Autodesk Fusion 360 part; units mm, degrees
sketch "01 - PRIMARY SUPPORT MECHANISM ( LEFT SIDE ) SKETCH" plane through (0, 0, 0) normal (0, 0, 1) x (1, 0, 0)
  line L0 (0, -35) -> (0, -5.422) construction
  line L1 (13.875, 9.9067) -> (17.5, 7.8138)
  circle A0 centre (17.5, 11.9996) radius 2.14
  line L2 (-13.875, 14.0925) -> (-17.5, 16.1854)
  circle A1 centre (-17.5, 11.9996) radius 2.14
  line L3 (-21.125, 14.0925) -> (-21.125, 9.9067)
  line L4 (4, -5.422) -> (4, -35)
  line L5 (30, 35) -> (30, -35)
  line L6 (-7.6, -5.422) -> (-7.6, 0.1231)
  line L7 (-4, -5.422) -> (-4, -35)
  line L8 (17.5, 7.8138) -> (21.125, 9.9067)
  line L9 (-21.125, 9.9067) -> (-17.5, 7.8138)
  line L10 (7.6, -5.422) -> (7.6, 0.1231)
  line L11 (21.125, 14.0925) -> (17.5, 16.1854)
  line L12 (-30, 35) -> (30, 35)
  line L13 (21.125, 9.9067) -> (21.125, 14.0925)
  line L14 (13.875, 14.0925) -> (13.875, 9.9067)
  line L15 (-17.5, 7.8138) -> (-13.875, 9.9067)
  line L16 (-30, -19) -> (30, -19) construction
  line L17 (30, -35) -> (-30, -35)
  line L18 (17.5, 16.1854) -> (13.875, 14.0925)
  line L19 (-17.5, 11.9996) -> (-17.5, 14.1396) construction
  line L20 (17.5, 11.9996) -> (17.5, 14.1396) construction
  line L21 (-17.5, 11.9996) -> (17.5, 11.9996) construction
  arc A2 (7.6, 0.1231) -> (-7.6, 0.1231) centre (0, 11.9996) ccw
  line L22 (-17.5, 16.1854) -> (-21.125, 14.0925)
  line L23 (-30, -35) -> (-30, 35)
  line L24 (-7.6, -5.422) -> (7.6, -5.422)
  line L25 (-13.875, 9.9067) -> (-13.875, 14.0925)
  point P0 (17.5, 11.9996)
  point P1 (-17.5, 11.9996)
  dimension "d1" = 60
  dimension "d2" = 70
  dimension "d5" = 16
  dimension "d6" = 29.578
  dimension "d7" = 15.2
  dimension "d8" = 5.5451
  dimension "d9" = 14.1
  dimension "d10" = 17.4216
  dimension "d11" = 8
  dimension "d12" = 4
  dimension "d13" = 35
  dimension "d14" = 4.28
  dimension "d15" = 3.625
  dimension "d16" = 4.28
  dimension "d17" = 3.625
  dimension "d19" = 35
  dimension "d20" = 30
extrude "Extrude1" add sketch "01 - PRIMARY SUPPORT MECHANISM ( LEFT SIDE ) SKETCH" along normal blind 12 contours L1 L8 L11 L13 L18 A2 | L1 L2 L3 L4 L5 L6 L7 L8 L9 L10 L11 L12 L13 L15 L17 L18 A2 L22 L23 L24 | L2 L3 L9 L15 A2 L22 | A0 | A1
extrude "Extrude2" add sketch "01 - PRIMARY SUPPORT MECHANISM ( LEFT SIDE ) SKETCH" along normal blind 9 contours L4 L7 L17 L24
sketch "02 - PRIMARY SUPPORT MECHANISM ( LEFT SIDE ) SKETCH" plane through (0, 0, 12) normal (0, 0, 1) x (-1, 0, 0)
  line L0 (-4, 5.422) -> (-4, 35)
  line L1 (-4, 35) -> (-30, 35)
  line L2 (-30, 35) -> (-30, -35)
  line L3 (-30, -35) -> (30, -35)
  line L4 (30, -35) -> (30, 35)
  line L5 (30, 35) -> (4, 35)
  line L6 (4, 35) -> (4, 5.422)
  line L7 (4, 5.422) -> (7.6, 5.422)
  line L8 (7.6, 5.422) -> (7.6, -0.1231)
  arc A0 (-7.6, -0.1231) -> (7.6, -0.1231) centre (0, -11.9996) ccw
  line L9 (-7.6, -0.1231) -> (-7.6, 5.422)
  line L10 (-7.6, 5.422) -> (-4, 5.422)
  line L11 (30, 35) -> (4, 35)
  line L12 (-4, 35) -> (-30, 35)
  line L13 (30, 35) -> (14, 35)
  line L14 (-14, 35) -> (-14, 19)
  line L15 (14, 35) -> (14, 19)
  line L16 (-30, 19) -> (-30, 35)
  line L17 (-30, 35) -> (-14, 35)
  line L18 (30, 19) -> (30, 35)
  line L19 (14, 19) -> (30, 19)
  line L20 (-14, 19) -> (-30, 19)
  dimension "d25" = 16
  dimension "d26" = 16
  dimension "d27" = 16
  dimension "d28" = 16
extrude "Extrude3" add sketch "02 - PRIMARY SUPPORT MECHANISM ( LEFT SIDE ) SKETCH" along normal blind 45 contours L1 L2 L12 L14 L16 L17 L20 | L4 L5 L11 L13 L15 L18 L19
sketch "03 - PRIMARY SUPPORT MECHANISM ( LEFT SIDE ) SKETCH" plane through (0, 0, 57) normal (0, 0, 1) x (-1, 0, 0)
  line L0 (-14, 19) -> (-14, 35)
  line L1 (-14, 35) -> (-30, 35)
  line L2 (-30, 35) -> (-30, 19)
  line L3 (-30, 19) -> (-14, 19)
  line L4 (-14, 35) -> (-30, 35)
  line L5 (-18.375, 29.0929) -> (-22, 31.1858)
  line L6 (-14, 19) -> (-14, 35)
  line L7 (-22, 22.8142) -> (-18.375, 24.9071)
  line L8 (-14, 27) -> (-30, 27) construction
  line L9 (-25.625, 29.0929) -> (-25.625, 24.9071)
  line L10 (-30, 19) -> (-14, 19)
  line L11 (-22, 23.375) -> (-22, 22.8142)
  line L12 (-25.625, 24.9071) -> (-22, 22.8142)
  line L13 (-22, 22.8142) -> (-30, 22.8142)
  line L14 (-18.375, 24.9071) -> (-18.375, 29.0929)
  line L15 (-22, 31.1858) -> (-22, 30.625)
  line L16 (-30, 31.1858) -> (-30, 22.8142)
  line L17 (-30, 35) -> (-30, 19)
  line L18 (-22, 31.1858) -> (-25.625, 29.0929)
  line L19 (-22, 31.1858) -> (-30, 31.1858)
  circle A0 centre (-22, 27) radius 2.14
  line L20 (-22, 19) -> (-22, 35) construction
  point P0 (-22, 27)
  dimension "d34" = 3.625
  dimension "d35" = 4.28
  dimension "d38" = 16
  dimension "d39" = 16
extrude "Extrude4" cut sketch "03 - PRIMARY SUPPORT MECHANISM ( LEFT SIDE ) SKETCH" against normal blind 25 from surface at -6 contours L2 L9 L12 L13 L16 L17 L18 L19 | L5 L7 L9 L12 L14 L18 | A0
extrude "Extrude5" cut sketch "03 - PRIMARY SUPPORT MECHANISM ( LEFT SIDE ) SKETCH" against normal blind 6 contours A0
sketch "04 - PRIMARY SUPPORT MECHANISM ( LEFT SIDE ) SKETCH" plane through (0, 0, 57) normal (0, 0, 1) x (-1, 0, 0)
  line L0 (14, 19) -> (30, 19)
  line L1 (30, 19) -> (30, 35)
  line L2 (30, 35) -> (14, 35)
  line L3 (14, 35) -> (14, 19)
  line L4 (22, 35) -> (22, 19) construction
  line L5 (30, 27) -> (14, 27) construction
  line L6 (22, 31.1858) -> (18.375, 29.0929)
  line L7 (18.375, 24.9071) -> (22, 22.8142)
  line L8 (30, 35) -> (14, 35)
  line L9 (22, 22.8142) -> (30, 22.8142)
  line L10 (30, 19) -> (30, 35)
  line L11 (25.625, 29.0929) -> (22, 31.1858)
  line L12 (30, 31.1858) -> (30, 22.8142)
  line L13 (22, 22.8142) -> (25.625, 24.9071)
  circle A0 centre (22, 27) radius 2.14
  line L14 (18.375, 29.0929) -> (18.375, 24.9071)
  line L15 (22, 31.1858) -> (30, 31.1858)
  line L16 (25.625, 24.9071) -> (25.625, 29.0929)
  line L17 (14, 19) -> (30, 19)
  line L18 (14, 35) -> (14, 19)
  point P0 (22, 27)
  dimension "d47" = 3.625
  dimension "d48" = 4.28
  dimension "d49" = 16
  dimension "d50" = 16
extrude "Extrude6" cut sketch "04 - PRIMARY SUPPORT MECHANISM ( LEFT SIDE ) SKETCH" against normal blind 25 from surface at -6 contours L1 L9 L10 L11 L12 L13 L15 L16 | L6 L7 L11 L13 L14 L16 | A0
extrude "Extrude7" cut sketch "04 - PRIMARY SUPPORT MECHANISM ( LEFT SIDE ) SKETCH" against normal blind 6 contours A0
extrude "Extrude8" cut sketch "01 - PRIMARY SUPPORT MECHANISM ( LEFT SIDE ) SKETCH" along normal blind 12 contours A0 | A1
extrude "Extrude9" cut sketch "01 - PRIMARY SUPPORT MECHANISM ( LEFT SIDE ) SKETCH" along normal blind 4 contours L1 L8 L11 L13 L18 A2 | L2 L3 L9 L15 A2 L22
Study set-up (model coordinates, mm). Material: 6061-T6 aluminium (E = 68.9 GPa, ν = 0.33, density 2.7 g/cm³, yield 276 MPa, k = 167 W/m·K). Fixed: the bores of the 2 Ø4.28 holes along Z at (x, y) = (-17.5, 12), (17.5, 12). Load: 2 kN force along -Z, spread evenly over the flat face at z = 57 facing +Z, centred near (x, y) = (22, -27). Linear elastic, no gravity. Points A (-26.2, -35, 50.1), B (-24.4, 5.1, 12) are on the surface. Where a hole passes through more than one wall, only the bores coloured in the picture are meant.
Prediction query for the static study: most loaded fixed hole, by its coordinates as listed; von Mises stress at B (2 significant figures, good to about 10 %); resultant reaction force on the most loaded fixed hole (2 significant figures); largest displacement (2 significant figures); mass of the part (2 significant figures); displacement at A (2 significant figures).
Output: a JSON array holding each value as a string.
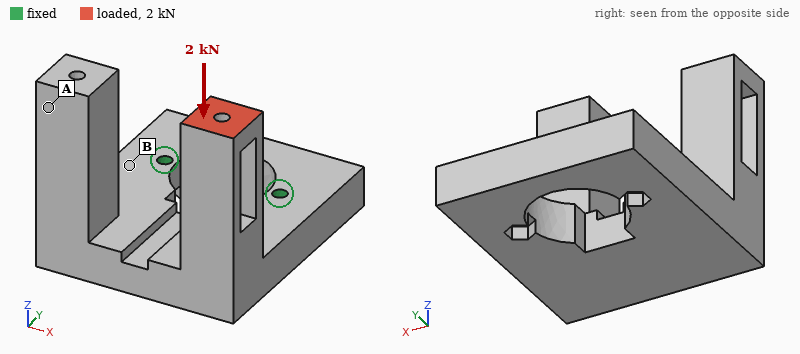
["(17.5, 12)", "57 MPa", "1.9 kN", "0.52 mm", "160 g", "0.31 mm"]
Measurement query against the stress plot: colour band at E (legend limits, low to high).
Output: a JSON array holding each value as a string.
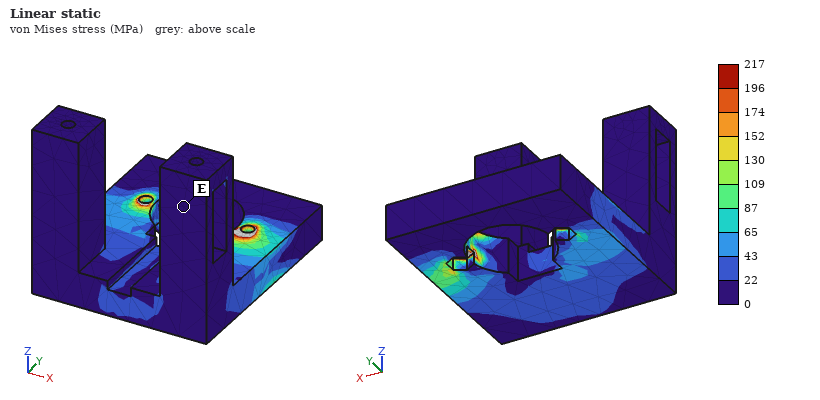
["0 to 22 MPa"]
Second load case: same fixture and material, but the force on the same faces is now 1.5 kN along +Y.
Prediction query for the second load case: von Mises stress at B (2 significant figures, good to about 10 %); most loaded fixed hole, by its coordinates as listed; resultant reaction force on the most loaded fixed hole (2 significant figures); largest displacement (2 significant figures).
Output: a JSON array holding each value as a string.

["72 MPa", "(17.5, 12)", "1.7 kN", "0.92 mm"]
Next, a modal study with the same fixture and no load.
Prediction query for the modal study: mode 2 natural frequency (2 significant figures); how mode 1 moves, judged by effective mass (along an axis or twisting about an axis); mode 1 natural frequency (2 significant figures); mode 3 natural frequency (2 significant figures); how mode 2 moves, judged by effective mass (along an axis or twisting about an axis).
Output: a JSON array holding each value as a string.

["2100 Hz", "along Z", "1300 Hz", "3000 Hz", "along X"]
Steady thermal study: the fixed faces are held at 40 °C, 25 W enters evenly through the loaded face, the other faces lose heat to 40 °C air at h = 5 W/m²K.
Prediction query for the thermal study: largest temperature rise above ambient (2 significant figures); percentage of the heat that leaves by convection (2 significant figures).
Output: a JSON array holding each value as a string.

["53 K", "4.3 %"]
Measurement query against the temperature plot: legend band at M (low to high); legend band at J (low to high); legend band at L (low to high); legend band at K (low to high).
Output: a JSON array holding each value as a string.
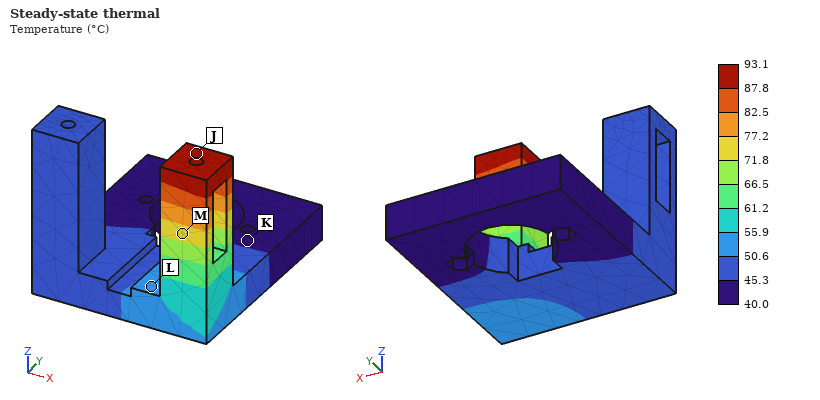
["71.8 to 77.2 °C", "87.8 to 93.1 °C", "50.6 to 55.9 °C", "40.0 to 45.3 °C"]
